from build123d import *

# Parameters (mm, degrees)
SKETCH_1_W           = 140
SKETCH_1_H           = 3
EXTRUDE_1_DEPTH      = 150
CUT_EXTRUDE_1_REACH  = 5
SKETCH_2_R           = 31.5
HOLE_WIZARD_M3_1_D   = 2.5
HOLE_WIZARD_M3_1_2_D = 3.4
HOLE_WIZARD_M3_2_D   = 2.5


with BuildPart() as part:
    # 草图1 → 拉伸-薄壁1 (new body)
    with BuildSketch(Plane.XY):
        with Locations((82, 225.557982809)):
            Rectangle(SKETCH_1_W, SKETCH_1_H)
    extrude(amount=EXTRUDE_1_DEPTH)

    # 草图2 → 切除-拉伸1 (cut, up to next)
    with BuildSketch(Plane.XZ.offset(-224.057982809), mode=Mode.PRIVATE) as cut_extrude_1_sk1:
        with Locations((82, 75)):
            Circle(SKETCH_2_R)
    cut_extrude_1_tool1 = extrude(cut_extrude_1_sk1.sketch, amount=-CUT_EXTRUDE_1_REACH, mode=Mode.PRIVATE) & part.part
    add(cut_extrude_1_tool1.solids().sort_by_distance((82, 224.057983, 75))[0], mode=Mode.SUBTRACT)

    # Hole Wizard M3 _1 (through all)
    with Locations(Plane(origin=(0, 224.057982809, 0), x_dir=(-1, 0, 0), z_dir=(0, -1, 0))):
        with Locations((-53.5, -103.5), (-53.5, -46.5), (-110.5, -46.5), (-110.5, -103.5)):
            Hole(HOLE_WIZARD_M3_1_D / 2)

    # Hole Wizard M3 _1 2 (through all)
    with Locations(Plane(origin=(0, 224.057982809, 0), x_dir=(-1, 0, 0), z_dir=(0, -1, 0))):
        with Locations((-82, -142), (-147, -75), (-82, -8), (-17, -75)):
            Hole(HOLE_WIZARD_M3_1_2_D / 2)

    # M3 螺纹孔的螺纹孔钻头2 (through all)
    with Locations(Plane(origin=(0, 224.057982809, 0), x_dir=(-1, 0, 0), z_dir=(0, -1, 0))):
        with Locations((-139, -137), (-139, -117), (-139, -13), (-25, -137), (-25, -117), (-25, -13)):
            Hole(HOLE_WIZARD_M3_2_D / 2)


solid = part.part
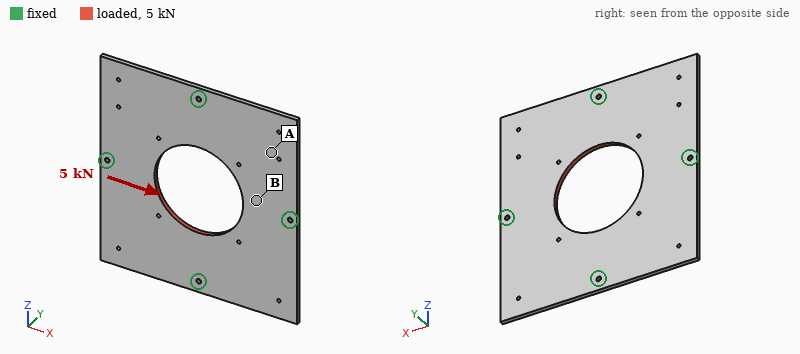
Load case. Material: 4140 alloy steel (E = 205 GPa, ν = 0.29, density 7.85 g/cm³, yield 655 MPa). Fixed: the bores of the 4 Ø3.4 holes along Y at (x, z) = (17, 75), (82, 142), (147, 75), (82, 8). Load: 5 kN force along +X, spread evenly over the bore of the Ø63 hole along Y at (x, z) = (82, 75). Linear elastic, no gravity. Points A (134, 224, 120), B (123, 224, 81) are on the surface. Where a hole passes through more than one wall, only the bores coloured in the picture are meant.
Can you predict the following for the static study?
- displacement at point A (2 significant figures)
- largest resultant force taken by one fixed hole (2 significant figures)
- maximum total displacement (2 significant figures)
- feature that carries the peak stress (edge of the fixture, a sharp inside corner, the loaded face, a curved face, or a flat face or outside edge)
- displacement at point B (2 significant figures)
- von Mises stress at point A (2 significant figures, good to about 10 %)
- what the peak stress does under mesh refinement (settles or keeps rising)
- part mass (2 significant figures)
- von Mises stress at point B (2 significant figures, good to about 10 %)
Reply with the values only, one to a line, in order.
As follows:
2.8 µm
1.3 kN
4.3 µm
edge of the fixture
2.7 µm
4.9 MPa
keeps rising
420 g
14 MPa
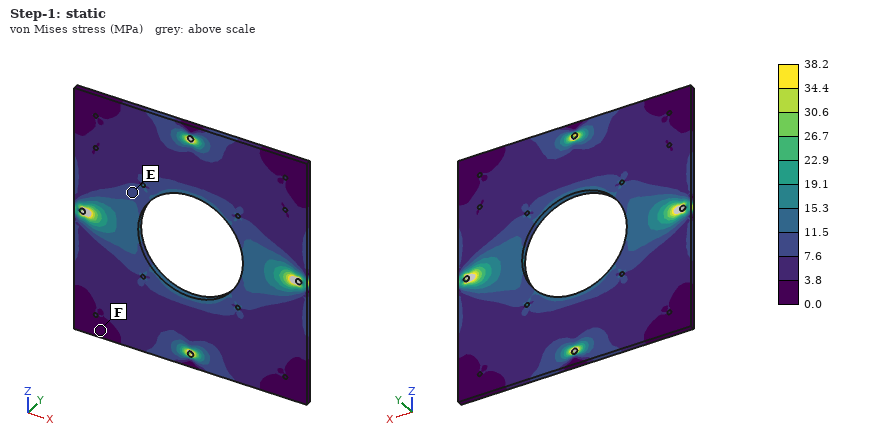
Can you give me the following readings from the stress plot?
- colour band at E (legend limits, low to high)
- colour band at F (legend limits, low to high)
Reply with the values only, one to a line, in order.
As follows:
7.6 to 11.5 MPa
0.0 to 3.8 MPa
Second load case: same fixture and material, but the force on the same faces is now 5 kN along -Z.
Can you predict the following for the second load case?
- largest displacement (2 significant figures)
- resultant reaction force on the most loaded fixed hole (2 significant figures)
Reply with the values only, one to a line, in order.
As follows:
4.3 µm
1.3 kN
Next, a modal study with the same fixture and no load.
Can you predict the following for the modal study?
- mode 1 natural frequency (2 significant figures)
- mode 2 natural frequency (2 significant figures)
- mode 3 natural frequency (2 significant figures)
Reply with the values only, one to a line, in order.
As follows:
830 Hz
890 Hz
900 Hz
